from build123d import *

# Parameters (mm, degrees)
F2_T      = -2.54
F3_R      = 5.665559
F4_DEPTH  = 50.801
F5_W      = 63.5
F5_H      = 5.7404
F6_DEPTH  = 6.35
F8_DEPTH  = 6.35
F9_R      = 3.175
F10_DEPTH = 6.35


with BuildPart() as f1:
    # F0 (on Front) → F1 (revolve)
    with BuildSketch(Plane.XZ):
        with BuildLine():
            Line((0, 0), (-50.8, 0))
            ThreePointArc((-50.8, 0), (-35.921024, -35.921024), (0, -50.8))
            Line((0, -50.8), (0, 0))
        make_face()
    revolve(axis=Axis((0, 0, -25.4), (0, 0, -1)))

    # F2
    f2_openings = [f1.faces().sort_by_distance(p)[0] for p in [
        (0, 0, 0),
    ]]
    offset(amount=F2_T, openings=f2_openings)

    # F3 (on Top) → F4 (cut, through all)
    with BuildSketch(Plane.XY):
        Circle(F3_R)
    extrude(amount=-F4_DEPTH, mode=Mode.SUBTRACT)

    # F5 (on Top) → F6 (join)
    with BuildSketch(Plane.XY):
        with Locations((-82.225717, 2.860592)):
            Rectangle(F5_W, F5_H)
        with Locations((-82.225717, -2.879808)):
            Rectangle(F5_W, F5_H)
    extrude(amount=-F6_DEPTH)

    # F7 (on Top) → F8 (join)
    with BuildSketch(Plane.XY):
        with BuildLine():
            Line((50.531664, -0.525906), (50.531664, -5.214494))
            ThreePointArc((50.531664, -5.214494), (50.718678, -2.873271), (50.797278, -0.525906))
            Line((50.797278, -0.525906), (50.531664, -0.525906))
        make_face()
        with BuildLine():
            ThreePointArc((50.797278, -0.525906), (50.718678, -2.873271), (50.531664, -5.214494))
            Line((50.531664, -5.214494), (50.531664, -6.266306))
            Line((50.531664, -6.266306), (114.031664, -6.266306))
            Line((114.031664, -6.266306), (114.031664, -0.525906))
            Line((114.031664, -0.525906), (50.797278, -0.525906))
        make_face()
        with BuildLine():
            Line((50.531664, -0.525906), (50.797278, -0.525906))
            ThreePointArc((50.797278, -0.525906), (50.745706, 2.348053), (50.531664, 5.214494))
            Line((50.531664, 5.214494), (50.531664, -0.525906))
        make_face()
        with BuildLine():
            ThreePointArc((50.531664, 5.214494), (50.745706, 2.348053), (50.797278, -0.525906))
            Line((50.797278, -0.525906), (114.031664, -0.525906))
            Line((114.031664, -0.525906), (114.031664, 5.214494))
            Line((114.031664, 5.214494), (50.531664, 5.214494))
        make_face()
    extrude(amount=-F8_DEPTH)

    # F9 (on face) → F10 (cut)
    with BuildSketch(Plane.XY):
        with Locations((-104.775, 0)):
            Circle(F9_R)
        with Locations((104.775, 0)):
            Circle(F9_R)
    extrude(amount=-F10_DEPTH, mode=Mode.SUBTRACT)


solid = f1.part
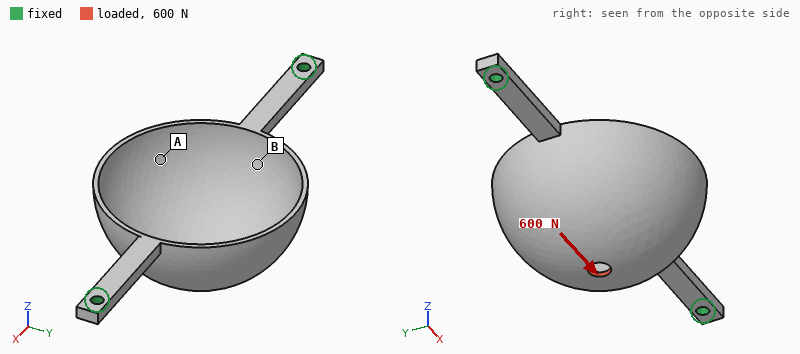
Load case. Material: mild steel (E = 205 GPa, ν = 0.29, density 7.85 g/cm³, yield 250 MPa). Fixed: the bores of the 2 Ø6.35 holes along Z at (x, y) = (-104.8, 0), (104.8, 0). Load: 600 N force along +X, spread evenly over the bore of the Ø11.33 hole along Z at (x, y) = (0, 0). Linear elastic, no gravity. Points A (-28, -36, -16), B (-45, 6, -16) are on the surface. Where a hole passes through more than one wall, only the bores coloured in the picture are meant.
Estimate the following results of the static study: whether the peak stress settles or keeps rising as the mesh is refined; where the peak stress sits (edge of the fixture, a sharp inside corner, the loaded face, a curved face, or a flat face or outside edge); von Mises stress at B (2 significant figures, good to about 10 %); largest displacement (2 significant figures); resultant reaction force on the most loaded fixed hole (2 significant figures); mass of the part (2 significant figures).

keeps rising
a sharp inside corner
20 MPa
84 µm
360 N
370 g
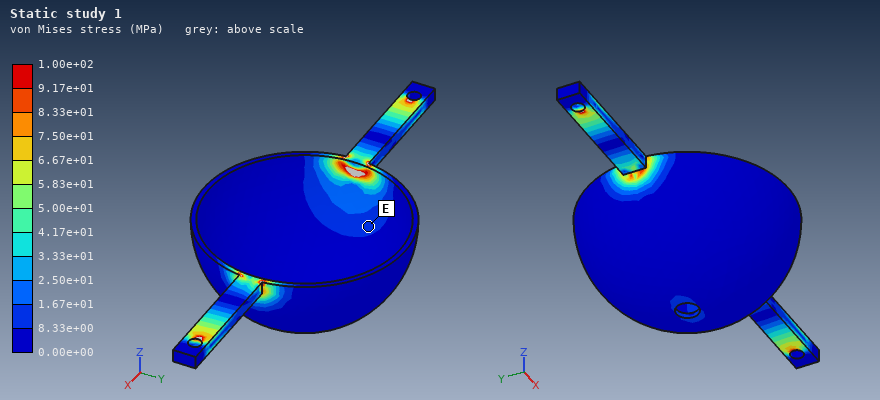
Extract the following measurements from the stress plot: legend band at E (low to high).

8.33e+00 to 1.67e+01 MPa
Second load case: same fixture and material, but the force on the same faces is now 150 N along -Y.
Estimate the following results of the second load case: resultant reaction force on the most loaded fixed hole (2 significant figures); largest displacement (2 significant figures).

75 N
0.22 mm
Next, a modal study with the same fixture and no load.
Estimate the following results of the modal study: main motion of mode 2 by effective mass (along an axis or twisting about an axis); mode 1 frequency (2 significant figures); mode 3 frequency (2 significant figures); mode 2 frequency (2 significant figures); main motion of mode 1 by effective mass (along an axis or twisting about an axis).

along Z
300 Hz
890 Hz
540 Hz
along Y
